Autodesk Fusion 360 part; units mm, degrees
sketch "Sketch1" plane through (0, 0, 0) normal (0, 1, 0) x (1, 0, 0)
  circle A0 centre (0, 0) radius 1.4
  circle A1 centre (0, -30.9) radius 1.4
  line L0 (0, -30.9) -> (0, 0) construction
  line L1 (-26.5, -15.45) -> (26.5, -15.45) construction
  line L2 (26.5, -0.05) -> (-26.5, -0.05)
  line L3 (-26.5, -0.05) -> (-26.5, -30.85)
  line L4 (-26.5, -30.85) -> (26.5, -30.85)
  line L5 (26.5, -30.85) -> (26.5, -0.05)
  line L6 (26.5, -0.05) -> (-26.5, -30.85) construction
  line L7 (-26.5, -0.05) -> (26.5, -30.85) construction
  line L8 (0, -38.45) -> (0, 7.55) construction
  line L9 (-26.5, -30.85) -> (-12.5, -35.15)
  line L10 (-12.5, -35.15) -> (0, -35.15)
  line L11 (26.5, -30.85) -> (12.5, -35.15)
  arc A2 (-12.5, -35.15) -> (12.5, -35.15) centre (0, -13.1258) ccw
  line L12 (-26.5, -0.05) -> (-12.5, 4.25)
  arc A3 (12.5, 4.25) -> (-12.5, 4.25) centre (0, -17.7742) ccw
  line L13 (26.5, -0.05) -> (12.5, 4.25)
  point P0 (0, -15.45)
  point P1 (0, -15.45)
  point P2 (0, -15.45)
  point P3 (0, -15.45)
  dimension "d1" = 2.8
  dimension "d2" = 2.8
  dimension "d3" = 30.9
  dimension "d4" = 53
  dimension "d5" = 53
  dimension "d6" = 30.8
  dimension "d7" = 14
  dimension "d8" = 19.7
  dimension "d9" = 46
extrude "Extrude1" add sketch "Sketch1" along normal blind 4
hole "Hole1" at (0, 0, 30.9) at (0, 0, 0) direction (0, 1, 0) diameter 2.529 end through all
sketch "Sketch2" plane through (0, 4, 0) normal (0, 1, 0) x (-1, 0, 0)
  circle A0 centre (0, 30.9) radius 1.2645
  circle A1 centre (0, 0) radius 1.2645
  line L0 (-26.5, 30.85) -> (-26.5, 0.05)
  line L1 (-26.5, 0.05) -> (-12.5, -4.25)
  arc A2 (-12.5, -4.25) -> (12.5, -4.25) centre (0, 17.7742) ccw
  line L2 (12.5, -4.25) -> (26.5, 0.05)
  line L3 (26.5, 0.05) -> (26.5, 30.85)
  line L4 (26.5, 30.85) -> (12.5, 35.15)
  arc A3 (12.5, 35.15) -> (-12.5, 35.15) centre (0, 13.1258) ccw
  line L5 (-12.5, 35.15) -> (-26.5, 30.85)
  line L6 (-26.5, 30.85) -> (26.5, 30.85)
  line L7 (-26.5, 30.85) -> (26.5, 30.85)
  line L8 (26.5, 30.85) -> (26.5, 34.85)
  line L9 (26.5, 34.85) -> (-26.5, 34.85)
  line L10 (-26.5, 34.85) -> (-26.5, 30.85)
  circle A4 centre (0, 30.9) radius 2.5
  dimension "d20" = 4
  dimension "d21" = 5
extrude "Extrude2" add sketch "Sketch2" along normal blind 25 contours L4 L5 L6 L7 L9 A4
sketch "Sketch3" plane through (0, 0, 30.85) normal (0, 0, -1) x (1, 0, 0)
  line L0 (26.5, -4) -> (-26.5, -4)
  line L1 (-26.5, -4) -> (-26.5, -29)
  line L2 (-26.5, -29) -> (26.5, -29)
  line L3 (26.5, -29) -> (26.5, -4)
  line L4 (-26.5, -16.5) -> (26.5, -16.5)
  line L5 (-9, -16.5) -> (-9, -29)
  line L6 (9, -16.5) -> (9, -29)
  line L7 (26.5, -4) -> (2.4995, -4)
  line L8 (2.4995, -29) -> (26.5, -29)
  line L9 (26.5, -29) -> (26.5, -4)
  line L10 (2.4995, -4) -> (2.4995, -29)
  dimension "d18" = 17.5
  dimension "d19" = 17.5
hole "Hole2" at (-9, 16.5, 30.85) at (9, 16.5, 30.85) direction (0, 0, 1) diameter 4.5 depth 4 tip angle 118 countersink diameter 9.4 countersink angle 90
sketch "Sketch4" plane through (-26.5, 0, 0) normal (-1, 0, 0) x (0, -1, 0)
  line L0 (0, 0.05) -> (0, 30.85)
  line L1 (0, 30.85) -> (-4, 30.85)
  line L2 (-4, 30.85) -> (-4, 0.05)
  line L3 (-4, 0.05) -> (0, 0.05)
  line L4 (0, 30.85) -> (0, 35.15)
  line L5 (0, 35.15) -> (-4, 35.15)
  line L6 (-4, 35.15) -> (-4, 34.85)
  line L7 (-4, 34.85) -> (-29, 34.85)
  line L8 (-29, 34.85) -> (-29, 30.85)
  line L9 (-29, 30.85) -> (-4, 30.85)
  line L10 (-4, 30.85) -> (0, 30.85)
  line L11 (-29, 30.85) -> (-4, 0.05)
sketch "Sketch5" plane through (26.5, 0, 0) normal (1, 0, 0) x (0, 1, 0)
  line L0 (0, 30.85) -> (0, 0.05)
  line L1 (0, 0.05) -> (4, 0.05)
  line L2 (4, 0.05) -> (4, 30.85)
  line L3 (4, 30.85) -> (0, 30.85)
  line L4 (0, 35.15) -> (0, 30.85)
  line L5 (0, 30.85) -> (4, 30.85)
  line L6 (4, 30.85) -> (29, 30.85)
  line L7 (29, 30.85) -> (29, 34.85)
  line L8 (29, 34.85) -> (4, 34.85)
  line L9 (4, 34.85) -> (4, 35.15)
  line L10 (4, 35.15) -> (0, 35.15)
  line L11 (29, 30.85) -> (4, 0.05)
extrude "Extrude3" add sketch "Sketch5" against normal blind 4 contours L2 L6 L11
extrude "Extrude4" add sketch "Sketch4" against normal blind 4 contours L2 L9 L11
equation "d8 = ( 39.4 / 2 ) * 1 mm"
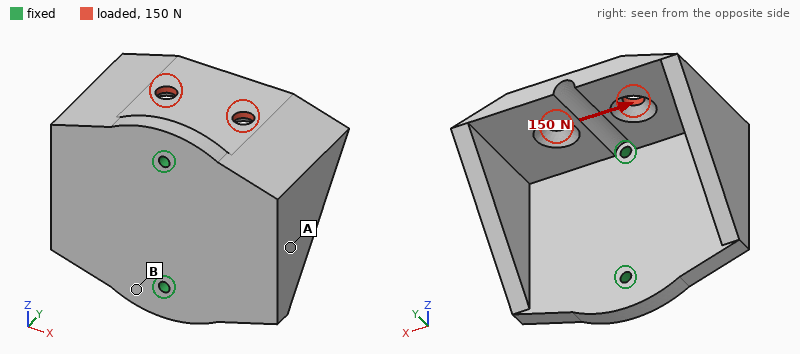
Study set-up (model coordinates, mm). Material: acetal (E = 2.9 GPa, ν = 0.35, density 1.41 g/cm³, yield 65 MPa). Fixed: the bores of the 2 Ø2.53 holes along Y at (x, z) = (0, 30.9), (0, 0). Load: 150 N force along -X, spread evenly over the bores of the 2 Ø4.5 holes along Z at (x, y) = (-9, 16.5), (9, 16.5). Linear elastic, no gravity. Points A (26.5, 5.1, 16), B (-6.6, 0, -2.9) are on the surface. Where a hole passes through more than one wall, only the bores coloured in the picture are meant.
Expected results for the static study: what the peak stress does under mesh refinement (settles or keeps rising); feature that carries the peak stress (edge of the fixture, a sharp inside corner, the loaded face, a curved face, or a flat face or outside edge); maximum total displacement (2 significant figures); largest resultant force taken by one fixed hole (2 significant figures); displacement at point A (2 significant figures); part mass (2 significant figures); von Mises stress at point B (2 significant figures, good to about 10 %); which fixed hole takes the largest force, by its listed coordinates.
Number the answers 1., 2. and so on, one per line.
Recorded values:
1. keeps rising
2. edge of the fixture
3. 0.76 mm
4. 160 N
5. 0.42 mm
6. 21 g
7. 5.3 MPa
8. (0, 30.9)
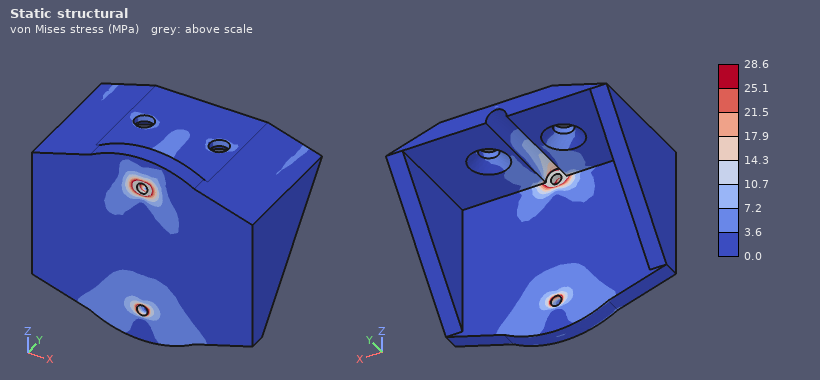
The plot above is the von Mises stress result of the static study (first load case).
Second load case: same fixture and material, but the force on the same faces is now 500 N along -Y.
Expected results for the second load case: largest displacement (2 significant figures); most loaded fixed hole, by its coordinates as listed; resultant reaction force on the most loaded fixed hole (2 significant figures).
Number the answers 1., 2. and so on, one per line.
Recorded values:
1. 0.31 mm
2. (0, 30.9)
3. 530 N
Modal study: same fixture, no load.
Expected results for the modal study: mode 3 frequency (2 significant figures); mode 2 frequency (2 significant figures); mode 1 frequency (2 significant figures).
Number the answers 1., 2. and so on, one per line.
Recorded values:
1. 1400 Hz
2. 1200 Hz
3. 660 Hz
